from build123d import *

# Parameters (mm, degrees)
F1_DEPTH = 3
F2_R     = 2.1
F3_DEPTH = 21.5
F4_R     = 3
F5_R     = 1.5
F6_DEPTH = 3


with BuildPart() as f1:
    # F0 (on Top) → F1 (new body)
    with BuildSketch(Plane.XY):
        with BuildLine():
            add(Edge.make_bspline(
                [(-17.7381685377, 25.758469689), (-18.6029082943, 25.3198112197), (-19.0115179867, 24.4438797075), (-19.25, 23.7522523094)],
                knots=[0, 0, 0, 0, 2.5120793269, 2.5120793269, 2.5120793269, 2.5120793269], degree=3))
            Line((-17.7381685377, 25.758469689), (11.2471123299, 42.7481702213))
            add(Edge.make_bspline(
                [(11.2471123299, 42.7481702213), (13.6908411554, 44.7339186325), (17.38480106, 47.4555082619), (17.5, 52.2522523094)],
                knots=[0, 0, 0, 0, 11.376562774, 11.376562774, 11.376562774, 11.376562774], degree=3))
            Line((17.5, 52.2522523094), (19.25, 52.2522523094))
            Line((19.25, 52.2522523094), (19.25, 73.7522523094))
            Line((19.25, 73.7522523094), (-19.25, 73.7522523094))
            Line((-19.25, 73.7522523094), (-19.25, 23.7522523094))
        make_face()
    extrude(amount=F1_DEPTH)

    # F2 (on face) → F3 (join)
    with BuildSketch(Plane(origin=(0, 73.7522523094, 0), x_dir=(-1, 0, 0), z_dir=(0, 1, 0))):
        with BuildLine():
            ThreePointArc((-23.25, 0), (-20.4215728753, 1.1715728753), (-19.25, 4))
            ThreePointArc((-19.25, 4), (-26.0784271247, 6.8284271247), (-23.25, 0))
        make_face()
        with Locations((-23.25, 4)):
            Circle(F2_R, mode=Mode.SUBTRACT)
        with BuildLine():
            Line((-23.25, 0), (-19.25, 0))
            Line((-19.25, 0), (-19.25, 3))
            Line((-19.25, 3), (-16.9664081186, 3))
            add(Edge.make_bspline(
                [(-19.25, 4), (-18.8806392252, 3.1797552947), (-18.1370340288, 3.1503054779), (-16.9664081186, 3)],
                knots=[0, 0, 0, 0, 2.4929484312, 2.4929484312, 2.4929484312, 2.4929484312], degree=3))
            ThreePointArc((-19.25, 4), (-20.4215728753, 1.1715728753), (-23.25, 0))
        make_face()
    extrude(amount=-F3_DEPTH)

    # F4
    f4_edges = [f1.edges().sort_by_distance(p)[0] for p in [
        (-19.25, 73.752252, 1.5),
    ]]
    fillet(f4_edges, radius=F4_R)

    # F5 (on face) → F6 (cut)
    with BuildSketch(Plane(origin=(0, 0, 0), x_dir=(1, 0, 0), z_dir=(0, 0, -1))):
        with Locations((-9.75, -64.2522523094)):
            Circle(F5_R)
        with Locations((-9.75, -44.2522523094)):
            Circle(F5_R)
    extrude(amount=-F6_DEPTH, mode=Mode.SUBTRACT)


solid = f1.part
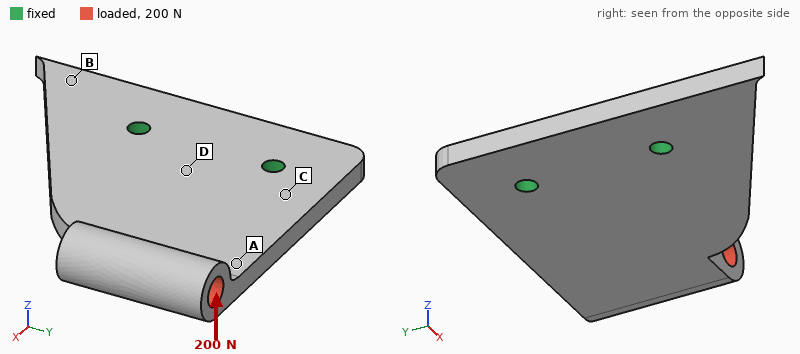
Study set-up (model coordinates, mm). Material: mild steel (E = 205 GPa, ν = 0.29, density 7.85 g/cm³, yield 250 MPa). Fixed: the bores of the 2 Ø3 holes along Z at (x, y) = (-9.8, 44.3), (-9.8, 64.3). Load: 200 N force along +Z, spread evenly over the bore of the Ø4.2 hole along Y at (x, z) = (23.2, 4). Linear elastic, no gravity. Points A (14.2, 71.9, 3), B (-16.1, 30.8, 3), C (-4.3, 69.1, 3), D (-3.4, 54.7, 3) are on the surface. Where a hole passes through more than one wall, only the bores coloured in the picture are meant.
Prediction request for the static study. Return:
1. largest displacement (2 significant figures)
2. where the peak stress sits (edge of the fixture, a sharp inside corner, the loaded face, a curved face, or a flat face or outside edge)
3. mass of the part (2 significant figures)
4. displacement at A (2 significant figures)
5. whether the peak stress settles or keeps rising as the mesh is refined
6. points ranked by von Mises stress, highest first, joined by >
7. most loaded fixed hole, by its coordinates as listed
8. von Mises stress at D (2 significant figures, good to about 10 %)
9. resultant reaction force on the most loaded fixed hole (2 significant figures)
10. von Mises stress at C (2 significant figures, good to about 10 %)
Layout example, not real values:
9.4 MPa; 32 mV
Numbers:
0.21 mm; edge of the fixture; 40 g; 0.11 mm; keeps rising; C > D > A > B; (-9.8, 64.3); 84 MPa; 170 N; 110 MPa
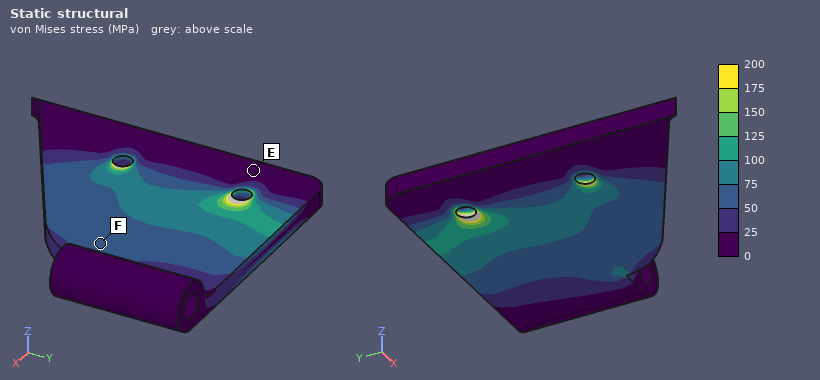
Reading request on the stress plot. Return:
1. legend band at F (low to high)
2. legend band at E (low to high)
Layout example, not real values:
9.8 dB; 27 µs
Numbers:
50 to 75 MPa; 0 to 25 MPa
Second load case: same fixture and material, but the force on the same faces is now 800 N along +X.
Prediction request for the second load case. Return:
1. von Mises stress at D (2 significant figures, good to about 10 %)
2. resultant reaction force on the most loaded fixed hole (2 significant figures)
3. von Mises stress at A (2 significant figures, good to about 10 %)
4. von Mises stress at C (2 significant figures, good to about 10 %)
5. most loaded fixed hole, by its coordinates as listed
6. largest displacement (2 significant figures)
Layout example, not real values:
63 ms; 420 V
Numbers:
37 MPa; 730 N; 63 MPa; 50 MPa; (-9.8, 64.3); 96 µm
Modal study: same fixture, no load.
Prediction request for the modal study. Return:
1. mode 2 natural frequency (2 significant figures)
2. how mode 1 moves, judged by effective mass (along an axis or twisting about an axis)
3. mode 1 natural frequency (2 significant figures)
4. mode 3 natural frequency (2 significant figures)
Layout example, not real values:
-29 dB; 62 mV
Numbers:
5900 Hz; along Z; 1800 Hz; 9400 Hz
